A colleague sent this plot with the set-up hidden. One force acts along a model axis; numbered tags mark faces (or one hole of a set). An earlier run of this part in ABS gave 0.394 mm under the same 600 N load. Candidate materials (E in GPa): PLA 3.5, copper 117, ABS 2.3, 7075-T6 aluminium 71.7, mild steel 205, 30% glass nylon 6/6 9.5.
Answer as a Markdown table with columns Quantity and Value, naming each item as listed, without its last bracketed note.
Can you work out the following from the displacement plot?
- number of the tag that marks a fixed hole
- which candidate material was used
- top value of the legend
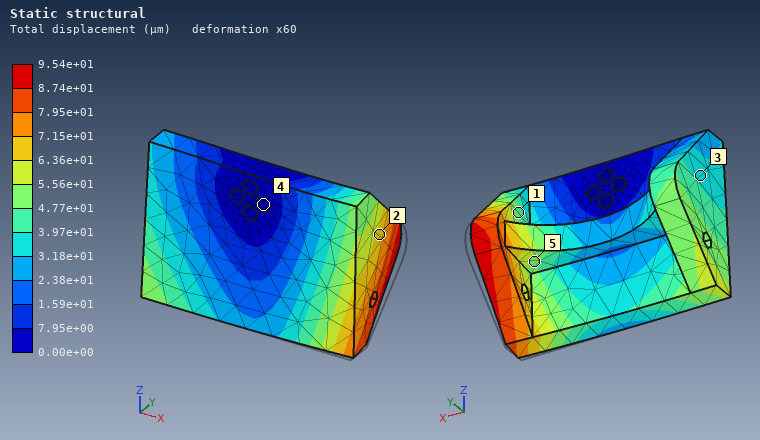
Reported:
| Quantity | Value |
|---|---|
| number of the tag that marks a fixed hole | 4 |
| which candidate material was used | 30% glass nylon 6/6 |
| top value of the legend | 9.54e+01 µm |
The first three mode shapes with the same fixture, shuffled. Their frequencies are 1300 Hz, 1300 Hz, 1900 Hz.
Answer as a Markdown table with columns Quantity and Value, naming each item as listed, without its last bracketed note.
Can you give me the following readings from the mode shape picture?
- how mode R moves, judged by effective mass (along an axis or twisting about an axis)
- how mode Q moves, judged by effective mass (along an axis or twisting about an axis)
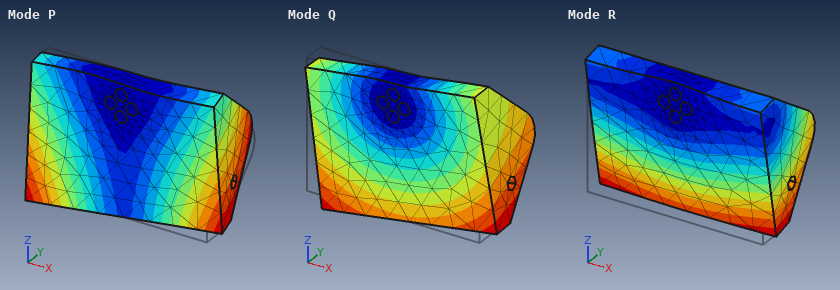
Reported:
| Quantity | Value |
|---|---|
| how mode R moves, judged by effective mass | along Y |
| how mode Q moves, judged by effective mass | along X |
